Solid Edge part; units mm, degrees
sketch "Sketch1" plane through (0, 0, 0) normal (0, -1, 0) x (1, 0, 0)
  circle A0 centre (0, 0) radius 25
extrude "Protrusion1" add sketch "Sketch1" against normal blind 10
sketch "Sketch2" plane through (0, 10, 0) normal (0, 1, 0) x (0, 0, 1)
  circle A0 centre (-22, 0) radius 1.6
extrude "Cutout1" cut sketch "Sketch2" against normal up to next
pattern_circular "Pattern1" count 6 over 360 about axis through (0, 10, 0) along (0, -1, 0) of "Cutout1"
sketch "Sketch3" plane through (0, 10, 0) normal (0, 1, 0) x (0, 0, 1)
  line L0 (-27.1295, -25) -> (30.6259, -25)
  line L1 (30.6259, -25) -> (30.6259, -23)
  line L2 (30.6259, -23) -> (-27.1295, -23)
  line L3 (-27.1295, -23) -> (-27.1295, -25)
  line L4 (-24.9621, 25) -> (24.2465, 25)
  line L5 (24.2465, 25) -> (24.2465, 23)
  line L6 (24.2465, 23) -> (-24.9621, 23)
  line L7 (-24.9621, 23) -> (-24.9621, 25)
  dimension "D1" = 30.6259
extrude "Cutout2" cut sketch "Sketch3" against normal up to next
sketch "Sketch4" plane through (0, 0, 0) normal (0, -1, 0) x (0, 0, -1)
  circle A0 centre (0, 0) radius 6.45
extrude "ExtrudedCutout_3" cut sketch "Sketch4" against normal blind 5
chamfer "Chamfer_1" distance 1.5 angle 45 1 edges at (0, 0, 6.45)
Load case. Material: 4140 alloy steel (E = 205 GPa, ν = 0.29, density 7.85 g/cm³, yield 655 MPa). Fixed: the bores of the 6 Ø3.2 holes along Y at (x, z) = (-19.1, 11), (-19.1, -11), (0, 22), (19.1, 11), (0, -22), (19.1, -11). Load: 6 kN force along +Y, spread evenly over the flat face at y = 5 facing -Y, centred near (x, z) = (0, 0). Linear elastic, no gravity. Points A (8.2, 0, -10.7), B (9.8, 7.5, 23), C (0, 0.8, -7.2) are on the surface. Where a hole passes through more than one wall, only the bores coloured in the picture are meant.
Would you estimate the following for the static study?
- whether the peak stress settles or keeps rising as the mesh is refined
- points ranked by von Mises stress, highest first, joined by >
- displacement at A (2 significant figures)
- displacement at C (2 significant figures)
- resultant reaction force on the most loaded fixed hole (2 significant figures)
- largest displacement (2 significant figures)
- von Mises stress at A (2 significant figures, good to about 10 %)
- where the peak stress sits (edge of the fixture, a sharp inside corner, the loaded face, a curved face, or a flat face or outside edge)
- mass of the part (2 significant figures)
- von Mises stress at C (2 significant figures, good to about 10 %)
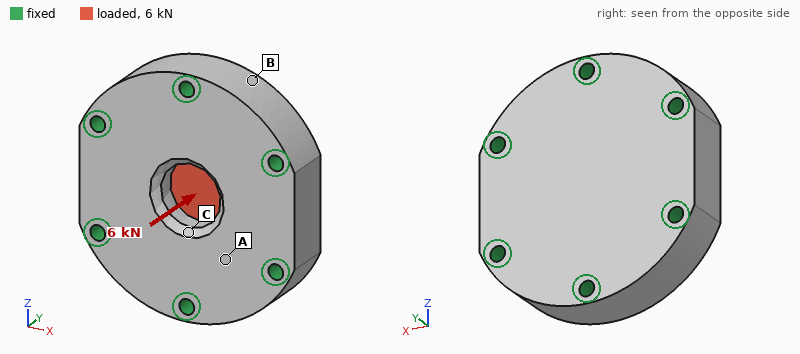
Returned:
keeps rising
C > A > B
3.0 µm
5.3 µm
1.1 kN
9.5 µm
27 MPa
edge of the fixture
140 g
47 MPa
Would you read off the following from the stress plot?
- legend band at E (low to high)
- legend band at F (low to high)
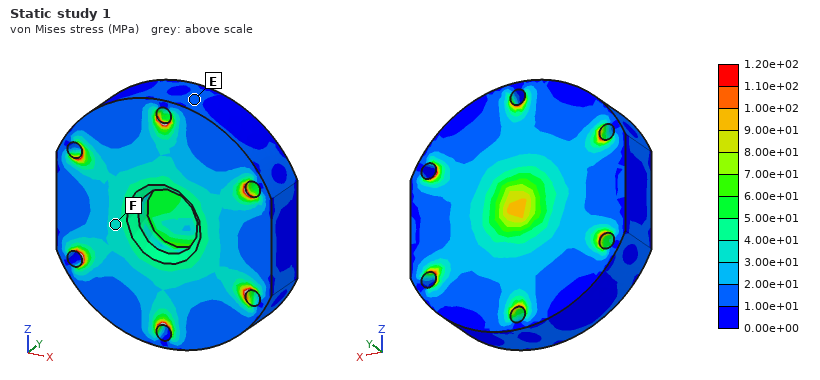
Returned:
1.00e+01 to 2.00e+01 MPa
3.00e+01 to 4.00e+01 MPa
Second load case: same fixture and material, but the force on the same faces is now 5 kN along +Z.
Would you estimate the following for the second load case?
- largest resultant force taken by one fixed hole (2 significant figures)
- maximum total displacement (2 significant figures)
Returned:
1.3 kN
2.9 µm
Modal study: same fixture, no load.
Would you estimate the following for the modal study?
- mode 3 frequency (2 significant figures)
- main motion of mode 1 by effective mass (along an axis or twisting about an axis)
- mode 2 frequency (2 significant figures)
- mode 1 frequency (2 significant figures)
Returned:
48 kHz
along Y
48 kHz
30 kHz
